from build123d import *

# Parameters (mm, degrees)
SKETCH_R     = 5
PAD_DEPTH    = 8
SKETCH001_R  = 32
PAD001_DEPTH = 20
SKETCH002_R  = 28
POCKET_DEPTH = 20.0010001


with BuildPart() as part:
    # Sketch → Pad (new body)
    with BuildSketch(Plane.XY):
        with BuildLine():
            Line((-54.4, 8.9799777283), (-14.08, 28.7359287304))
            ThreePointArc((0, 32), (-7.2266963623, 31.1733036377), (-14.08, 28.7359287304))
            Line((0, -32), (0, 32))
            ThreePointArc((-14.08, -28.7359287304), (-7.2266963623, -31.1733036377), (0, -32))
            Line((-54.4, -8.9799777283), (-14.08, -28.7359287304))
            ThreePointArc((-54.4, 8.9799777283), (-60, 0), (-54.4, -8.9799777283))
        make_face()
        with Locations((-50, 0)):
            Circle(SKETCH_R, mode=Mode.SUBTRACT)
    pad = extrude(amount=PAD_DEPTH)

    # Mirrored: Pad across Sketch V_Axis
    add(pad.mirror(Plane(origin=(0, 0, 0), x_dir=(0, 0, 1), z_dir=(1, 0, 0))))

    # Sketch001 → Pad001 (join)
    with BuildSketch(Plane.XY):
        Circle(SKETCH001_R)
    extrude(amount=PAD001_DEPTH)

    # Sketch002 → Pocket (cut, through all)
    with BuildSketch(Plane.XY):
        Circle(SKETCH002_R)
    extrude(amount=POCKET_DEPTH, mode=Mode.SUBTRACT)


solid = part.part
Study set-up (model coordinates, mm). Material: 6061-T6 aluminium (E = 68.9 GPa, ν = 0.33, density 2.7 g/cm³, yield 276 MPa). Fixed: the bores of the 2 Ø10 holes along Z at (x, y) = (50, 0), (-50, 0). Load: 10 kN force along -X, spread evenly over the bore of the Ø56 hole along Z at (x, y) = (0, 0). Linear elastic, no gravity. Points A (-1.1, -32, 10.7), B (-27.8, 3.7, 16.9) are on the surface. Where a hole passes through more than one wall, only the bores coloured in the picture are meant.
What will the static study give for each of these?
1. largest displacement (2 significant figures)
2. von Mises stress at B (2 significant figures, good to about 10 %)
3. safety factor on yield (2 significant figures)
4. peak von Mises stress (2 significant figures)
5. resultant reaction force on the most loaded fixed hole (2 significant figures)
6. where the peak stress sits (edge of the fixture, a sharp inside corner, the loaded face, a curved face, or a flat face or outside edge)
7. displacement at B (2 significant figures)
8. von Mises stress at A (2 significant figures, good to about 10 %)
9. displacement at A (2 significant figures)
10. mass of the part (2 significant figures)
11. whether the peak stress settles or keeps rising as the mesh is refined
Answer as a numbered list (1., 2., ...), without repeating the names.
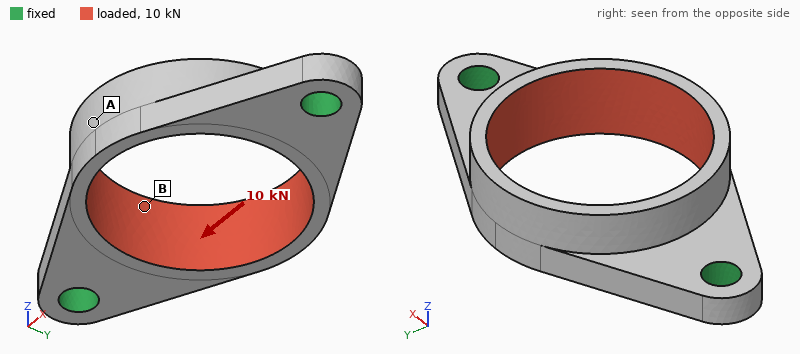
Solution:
1. 52 µm
2. 40 MPa
3. 3.6
4. 78 MPa
5. 5.1 kN
6. the loaded face
7. 13 µm
8. 14 MPa
9. 30 µm
10. 74 g
11. settles
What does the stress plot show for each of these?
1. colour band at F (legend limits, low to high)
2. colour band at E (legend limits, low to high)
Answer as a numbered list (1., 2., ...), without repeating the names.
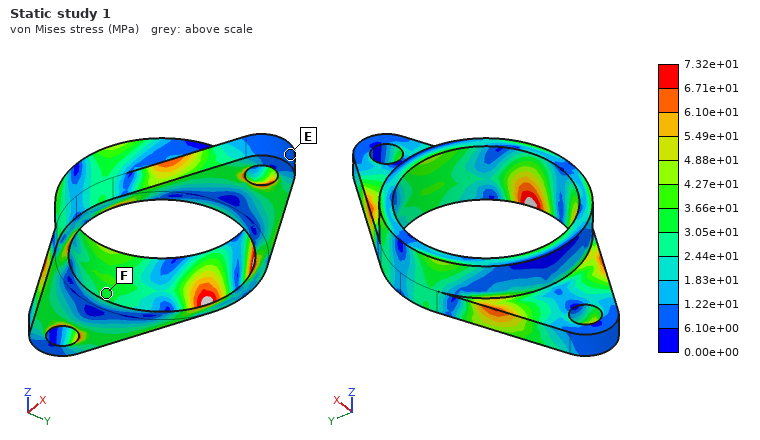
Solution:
1. 3.05e+01 to 3.66e+01 MPa
2. 6.10e+00 to 1.22e+01 MPa
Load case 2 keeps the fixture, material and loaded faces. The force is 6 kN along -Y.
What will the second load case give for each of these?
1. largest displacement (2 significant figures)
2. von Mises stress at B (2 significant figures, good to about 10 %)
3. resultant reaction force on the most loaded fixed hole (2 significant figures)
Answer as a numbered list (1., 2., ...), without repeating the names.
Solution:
1. 0.15 mm
2. 16 MPa
3. 3.0 kN
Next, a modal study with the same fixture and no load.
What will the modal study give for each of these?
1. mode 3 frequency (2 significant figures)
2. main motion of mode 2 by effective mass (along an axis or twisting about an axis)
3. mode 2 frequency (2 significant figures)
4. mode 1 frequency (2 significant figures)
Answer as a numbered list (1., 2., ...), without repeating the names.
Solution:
1. 6900 Hz
2. along Z
3. 4100 Hz
4. 3400 Hz
